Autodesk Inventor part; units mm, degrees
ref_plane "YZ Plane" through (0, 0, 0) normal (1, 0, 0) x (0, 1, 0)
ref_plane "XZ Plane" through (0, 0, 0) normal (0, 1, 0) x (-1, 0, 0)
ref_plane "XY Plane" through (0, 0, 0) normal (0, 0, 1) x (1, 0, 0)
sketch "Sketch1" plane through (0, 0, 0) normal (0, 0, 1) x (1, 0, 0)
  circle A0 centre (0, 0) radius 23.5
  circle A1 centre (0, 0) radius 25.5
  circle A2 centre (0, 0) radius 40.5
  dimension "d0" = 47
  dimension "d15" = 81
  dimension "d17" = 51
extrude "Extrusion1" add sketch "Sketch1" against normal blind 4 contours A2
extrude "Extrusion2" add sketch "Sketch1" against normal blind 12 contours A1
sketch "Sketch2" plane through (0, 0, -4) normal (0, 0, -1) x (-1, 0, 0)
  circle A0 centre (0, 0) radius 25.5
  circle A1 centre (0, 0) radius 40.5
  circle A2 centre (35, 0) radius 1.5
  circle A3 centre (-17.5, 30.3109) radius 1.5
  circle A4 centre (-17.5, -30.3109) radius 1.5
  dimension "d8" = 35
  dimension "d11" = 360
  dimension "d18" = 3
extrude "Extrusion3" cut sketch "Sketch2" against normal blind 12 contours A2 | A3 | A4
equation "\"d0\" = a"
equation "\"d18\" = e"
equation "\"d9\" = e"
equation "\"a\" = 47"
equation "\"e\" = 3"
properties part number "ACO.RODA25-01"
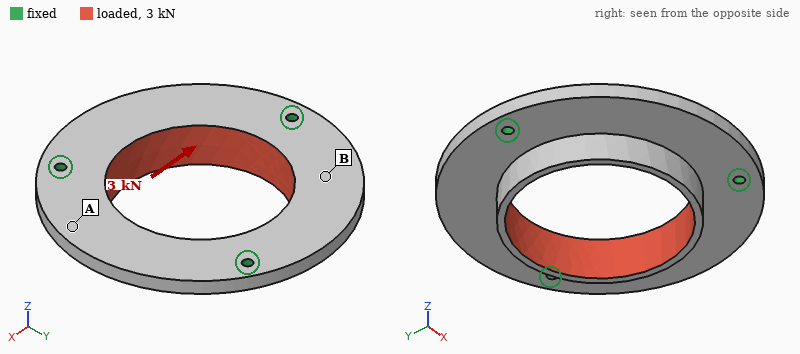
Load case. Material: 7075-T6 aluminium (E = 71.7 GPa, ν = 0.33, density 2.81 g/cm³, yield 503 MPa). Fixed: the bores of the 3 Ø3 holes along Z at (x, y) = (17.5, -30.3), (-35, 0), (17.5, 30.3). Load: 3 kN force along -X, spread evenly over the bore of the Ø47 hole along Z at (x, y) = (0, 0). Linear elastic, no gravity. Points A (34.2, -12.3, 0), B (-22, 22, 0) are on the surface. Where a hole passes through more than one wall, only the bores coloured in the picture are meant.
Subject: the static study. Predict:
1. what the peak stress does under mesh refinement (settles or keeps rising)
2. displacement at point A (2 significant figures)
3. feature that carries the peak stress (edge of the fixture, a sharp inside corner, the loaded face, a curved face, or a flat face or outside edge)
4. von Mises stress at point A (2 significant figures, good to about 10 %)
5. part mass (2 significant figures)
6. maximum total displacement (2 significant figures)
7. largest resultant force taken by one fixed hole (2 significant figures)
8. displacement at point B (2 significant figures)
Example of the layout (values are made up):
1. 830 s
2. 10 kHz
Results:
1. keeps rising
2. 31 µm
3. edge of the fixture
4. 15 MPa
5. 45 g
6. 46 µm
7. 1.2 kN
8. 14 µm
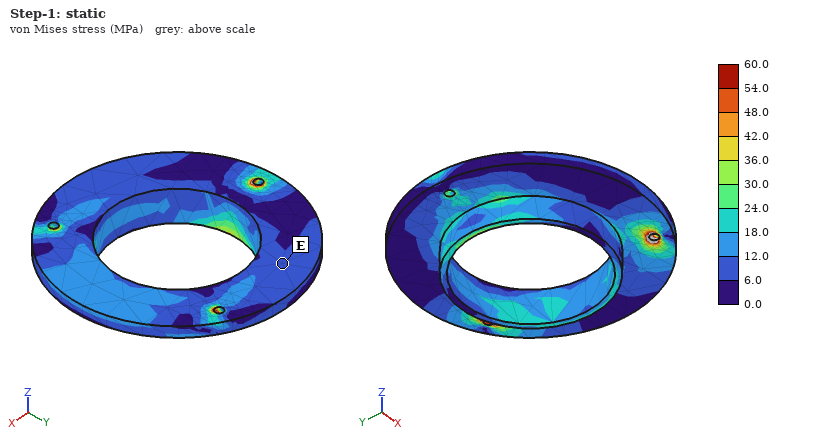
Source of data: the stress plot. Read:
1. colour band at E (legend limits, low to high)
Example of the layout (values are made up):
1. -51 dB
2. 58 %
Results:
1. 6.0 to 12.0 MPa
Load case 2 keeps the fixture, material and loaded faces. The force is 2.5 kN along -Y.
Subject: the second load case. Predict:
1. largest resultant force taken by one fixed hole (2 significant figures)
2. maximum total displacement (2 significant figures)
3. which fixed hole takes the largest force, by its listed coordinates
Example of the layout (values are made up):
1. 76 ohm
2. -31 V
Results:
1. 1.1 kN
2. 33 µm
3. (-35, 0)
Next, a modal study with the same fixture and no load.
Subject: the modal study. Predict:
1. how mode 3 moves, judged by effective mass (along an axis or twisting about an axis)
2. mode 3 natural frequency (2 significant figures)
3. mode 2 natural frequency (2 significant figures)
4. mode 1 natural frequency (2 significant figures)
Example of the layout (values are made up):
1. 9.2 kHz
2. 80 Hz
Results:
1. along Z
2. 4800 Hz
3. 3800 Hz
4. 3800 Hz
